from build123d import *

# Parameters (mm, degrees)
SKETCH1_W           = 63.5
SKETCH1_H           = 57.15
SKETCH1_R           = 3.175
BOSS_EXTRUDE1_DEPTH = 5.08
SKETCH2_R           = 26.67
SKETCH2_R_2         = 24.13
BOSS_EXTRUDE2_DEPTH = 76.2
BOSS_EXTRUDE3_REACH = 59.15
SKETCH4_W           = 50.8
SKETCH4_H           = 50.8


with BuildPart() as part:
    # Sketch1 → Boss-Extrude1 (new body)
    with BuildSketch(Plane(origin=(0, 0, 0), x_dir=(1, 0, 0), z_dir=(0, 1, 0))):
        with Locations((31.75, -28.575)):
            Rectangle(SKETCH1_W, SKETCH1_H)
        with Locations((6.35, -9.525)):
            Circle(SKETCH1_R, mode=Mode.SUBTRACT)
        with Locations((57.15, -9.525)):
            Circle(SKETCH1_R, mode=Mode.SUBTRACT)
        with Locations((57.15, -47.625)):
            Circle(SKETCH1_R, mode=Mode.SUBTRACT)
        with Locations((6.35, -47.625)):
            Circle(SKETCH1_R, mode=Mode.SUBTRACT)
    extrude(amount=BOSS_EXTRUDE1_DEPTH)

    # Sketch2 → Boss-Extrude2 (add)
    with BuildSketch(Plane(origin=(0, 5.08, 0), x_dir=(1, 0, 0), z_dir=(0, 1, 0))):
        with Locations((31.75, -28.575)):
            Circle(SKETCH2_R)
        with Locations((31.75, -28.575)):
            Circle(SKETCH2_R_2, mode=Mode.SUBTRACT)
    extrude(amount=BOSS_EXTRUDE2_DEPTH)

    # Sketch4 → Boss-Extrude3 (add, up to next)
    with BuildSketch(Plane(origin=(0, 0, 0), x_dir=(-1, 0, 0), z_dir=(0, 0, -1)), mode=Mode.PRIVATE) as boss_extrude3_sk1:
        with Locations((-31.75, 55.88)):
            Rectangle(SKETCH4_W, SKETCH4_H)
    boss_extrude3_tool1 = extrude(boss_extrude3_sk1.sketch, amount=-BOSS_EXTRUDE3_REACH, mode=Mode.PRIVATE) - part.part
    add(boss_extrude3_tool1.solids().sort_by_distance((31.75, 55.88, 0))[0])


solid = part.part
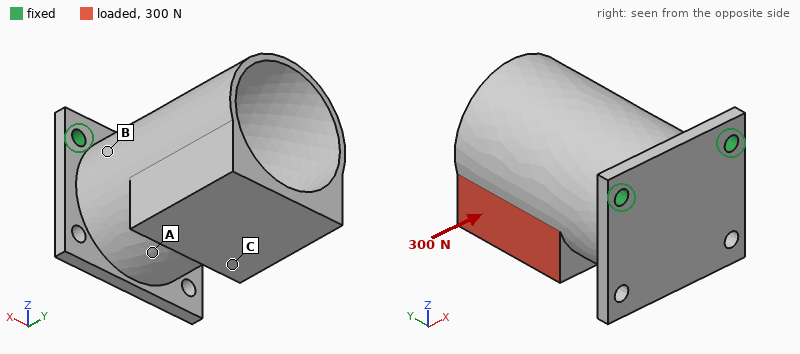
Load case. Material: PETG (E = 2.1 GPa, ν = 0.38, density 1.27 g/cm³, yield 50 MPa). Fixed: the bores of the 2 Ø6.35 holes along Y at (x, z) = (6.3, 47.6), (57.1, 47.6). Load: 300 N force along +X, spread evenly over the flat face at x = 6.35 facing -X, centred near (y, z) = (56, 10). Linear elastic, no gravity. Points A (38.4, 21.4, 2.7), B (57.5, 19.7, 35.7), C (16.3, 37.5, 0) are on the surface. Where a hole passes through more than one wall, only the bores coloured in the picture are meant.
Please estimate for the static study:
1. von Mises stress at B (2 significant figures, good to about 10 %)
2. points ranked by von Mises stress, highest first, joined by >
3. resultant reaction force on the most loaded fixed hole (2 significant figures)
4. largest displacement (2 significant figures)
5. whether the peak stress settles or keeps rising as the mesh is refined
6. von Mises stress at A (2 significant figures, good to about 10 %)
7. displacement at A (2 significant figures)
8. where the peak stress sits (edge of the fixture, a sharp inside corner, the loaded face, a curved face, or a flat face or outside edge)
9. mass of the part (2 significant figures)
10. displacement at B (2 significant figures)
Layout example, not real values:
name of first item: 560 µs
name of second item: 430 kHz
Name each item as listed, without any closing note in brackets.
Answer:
von Mises stress at B: 4.6 MPa
points ranked by von Mises stress, highest first, joined by >: B > A > C
resultant reaction force on the most loaded fixed hole: 430 N
largest displacement: 1.2 mm
whether the peak stress settles or keeps rising as the mesh is refined: keeps rising
von Mises stress at A: 2.5 MPa
displacement at A: 0.33 mm
where the peak stress sits: edge of the fixture
mass of the part: 84 g
displacement at B: 0.18 mm
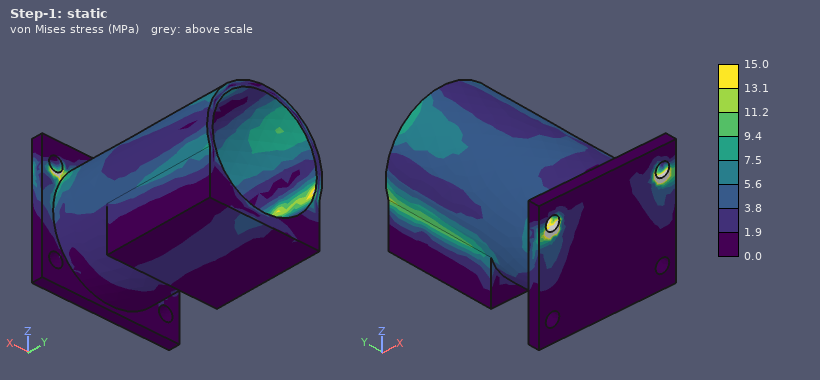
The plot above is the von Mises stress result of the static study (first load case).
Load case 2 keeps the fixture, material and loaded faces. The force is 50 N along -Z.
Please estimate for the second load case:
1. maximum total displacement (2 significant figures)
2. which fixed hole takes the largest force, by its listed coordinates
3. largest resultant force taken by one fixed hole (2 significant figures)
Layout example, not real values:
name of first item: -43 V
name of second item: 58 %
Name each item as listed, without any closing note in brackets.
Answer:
maximum total displacement: 1.2 mm
which fixed hole takes the largest force, by its listed coordinates: (6.3, 47.6)
largest resultant force taken by one fixed hole: 50 N
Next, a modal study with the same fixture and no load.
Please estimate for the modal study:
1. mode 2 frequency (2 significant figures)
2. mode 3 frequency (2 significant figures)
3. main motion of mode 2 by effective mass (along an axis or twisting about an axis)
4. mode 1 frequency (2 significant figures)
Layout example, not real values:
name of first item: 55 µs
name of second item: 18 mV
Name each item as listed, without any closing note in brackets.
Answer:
mode 2 frequency: 490 Hz
mode 3 frequency: 970 Hz
main motion of mode 2 by effective mass: along X
mode 1 frequency: 150 Hz
